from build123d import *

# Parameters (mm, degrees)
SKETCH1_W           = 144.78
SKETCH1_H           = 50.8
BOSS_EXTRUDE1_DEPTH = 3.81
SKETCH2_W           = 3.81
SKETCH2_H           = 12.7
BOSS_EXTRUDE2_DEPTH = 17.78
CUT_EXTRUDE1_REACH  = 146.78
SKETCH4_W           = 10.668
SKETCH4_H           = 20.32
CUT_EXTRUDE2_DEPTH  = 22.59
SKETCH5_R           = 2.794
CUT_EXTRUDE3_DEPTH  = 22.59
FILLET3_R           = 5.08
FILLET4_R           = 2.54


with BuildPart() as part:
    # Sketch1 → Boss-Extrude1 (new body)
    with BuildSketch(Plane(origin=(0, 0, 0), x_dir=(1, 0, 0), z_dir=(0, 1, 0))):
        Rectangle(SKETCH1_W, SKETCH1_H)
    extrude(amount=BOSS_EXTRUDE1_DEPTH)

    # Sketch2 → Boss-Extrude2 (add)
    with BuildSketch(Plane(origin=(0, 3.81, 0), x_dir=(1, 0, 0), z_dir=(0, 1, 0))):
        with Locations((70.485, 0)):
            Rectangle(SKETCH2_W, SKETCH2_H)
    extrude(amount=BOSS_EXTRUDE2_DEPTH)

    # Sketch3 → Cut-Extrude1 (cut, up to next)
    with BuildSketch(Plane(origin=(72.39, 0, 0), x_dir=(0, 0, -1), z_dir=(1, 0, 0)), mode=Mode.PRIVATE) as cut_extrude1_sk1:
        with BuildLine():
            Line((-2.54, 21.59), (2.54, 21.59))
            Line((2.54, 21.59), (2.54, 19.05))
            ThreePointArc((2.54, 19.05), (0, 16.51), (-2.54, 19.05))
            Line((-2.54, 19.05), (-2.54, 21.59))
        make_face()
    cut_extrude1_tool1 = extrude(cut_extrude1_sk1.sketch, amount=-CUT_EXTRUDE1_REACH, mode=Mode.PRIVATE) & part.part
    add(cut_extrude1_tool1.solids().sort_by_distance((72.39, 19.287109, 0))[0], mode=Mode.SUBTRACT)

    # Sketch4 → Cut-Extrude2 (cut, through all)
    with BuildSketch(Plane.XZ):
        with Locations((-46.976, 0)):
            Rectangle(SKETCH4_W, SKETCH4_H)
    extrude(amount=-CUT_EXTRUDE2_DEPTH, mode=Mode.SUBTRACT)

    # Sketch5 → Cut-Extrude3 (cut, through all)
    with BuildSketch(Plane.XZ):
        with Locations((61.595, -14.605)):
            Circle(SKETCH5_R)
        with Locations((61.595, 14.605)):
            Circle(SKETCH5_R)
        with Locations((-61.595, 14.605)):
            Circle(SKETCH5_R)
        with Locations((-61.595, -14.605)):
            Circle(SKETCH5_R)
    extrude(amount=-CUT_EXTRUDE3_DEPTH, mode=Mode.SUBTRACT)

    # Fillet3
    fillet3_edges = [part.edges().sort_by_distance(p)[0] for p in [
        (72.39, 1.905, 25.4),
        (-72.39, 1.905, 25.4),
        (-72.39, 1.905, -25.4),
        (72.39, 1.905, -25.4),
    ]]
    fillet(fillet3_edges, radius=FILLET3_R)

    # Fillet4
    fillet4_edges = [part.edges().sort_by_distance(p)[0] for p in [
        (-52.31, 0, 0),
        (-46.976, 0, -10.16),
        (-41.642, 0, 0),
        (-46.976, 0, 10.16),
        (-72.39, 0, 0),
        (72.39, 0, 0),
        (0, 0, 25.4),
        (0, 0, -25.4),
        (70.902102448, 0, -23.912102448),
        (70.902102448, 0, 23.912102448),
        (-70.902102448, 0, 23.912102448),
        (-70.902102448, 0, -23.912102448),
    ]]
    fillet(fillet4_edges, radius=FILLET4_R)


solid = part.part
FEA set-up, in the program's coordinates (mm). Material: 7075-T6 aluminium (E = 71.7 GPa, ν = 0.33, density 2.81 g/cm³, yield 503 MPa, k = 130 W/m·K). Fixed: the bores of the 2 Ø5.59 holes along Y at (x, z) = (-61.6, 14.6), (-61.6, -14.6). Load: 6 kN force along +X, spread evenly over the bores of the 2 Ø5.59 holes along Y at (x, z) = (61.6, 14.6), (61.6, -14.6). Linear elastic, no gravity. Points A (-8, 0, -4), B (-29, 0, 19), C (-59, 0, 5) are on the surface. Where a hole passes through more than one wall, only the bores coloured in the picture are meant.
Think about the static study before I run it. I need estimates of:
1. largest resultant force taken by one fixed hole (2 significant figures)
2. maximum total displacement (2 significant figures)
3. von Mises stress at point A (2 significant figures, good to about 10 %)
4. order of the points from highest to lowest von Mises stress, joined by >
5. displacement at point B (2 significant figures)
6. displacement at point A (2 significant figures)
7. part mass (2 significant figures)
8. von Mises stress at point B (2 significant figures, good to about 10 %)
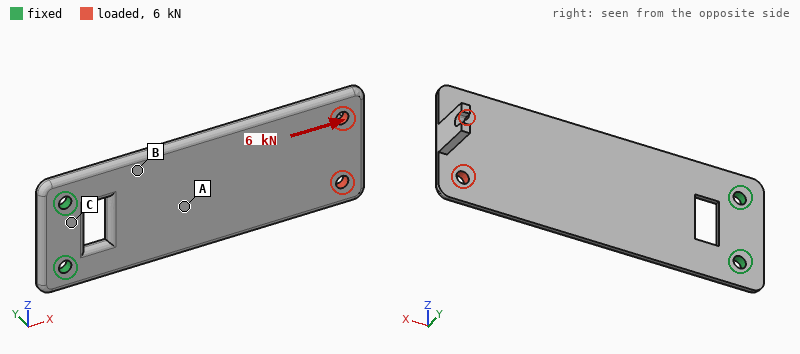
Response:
3.0 kN
0.17 mm
29 MPa
B > A > C
0.030 mm
0.055 mm
76 g
46 MPa
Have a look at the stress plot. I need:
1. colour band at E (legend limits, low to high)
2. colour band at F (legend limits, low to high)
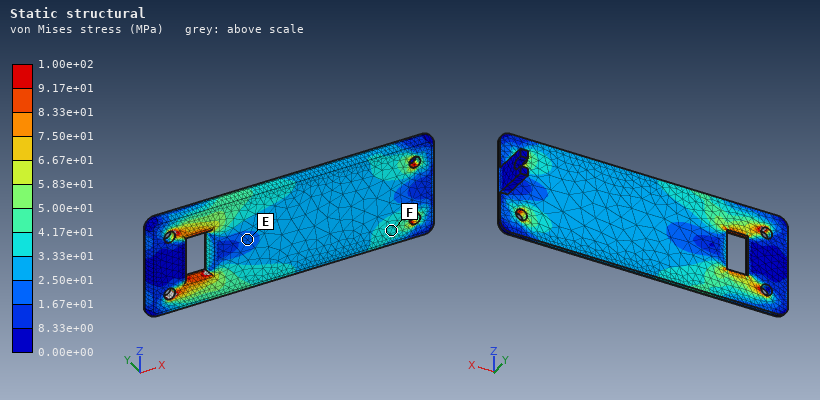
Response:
1.67e+01 to 2.50e+01 MPa
3.33e+01 to 4.17e+01 MPa
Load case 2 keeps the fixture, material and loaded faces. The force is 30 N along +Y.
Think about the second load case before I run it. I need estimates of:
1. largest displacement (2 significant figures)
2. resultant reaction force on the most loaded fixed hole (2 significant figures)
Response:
1.7 mm
17 N
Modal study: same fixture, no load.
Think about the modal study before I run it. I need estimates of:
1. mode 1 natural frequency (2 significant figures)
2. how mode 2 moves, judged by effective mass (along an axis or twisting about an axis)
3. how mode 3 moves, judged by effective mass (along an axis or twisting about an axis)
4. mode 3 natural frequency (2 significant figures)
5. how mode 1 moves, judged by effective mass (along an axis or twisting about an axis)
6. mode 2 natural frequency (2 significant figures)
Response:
140 Hz
twisting about X
along Y
1000 Hz
along Y
910 Hz
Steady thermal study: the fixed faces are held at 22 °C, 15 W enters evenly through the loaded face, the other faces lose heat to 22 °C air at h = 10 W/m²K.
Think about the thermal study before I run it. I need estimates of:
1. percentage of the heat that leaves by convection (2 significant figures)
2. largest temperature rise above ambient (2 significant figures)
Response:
35 %
65 K
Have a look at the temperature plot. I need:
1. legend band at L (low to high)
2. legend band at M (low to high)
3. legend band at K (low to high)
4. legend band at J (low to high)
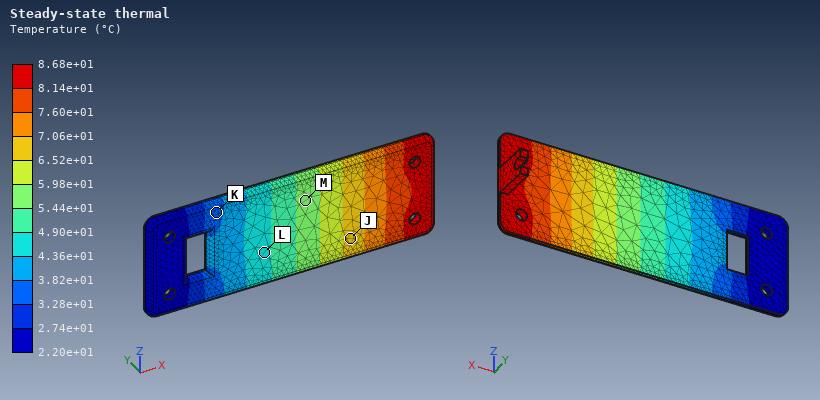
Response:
4.36e+01 to 4.90e+01 °C
5.44e+01 to 5.98e+01 °C
3.28e+01 to 3.82e+01 °C
6.52e+01 to 7.06e+01 °C
